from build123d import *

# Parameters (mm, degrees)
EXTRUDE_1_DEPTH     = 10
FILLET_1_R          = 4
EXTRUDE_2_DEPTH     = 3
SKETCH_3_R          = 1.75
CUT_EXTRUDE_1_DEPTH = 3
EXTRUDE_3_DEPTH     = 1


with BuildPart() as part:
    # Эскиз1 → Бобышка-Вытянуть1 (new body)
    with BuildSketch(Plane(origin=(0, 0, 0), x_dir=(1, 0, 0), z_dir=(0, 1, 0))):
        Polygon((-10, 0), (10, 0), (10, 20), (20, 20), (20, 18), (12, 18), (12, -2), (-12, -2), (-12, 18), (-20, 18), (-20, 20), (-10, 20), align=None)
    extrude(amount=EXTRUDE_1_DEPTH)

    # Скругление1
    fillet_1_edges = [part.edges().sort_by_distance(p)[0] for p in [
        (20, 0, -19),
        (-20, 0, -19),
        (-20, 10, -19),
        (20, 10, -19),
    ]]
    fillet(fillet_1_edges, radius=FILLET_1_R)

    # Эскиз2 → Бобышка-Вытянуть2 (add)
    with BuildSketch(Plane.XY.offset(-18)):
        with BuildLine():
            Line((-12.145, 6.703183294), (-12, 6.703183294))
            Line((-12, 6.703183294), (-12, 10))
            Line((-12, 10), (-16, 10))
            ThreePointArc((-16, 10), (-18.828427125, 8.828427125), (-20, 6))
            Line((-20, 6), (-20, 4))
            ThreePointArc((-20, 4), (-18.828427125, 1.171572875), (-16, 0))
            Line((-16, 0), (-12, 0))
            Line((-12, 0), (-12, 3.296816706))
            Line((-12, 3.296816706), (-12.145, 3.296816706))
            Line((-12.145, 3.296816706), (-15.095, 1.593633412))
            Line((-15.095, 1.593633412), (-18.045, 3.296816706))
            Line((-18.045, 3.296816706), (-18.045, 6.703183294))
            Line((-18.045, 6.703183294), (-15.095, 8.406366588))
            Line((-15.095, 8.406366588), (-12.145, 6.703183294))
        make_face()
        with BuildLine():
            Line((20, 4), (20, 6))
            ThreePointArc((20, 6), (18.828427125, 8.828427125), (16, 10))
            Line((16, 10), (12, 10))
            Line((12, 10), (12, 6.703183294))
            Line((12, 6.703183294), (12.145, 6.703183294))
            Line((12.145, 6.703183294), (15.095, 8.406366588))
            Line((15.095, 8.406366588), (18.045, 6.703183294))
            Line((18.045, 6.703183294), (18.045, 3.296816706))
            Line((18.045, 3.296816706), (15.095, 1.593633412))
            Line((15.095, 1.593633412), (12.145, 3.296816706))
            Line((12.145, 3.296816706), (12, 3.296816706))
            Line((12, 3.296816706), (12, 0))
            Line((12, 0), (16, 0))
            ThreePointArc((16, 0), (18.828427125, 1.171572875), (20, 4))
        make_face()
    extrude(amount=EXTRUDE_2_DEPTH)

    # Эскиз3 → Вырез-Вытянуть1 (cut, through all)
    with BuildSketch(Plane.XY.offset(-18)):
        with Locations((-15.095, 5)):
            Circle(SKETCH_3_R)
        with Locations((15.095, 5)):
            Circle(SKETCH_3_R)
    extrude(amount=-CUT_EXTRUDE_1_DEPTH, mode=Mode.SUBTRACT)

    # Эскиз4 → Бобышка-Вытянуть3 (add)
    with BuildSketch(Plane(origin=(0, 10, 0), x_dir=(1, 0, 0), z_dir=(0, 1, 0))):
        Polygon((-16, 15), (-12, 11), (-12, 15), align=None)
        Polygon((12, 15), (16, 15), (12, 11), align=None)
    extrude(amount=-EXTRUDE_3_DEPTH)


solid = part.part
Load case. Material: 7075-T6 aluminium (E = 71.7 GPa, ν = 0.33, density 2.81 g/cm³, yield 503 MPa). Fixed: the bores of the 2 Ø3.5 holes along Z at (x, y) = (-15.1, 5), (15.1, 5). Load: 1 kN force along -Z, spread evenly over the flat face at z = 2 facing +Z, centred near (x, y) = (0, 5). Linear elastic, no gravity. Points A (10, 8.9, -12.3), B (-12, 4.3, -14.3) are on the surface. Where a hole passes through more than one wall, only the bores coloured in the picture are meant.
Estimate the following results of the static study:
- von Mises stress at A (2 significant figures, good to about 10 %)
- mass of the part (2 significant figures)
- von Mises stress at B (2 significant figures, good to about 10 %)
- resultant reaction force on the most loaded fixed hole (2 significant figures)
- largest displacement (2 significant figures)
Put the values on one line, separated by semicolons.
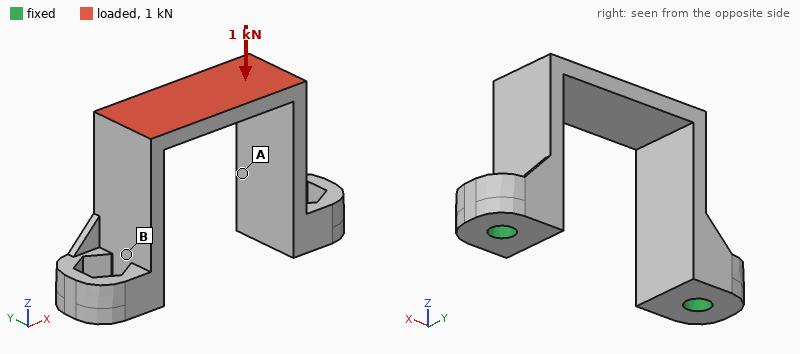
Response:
34 MPa; 5.1 g; 68 MPa; 520 N; 0.11 mm
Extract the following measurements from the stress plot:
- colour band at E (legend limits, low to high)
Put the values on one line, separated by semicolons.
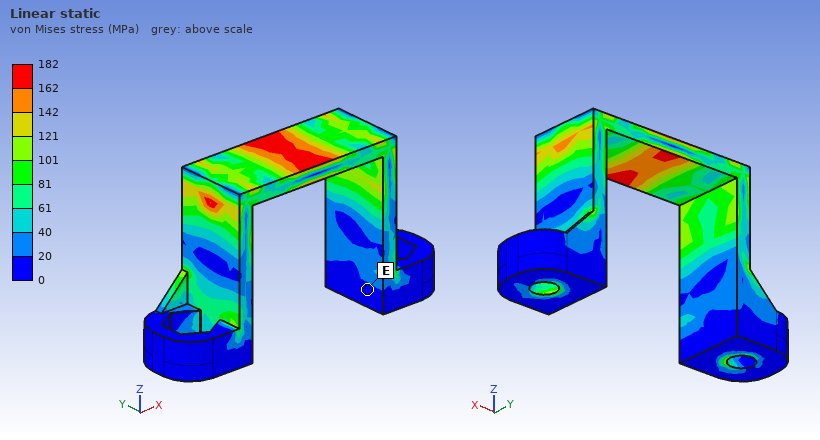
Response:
0 to 20 MPa
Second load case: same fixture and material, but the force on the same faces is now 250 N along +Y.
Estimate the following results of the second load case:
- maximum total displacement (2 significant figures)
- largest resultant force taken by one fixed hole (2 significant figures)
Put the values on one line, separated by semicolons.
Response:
0.11 mm; 130 N
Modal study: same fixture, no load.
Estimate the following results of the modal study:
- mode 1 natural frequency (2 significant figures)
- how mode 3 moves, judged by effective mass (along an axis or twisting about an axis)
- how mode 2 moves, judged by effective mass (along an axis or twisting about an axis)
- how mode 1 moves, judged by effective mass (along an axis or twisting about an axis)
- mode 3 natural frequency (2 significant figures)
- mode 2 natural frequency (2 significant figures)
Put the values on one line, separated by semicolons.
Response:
4700 Hz; twisting about Z; along Y; along X; 8300 Hz; 5900 Hz
